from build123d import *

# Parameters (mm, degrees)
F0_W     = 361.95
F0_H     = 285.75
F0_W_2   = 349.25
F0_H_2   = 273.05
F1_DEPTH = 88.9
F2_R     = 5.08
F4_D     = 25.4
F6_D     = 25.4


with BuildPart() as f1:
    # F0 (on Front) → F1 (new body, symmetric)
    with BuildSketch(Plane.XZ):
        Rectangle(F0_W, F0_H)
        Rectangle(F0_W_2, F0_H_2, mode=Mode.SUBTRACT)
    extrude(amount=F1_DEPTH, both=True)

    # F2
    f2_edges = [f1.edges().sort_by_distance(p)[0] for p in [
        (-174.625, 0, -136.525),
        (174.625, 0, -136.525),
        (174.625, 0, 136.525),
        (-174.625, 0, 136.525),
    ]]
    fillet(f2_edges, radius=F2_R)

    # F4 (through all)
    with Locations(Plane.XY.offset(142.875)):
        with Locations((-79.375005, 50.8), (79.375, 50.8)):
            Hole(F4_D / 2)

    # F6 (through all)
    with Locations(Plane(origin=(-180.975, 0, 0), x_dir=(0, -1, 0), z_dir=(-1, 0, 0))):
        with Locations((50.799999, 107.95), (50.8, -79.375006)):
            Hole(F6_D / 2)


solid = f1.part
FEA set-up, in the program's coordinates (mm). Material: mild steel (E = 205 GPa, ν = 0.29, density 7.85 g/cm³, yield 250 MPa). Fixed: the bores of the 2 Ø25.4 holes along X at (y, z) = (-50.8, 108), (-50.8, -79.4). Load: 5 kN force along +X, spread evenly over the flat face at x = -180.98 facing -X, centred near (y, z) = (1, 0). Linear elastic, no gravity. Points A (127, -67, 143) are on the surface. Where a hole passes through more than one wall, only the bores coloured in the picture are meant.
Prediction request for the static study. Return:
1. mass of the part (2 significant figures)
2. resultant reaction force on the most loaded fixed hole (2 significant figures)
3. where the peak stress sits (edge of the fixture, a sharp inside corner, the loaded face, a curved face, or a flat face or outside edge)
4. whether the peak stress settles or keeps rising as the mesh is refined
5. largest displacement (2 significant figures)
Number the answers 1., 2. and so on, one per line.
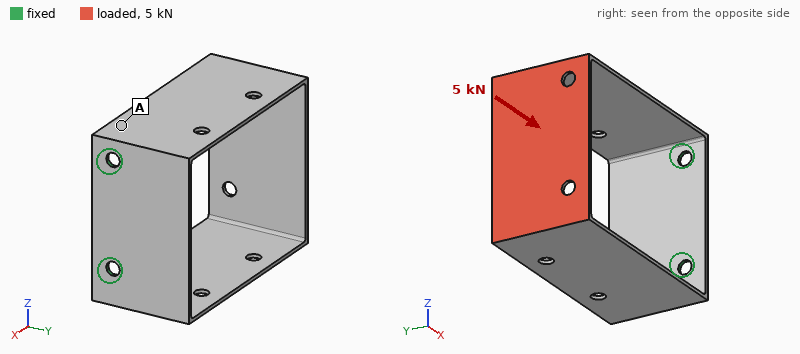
1. 11 kg
2. 2.6 kN
3. edge of the fixture
4. keeps rising
5. 2.1 mm
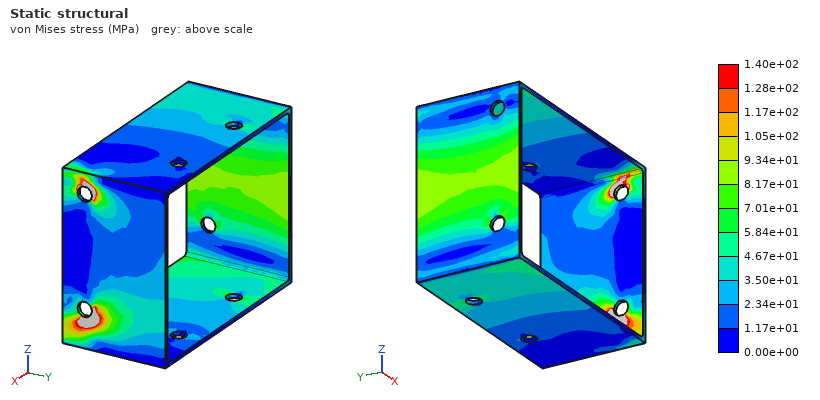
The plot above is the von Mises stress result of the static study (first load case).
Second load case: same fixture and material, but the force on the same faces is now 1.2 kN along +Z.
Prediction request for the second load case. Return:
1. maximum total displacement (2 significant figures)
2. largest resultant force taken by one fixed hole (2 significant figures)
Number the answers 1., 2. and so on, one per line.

1. 5.4 mm
2. 1.3 kN
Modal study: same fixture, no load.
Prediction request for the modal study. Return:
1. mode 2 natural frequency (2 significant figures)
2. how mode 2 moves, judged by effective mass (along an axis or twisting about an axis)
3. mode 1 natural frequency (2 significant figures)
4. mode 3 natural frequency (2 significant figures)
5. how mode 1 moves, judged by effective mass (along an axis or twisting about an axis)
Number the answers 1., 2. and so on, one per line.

1. 53 Hz
2. along Y
3. 35 Hz
4. 98 Hz
5. along Z
